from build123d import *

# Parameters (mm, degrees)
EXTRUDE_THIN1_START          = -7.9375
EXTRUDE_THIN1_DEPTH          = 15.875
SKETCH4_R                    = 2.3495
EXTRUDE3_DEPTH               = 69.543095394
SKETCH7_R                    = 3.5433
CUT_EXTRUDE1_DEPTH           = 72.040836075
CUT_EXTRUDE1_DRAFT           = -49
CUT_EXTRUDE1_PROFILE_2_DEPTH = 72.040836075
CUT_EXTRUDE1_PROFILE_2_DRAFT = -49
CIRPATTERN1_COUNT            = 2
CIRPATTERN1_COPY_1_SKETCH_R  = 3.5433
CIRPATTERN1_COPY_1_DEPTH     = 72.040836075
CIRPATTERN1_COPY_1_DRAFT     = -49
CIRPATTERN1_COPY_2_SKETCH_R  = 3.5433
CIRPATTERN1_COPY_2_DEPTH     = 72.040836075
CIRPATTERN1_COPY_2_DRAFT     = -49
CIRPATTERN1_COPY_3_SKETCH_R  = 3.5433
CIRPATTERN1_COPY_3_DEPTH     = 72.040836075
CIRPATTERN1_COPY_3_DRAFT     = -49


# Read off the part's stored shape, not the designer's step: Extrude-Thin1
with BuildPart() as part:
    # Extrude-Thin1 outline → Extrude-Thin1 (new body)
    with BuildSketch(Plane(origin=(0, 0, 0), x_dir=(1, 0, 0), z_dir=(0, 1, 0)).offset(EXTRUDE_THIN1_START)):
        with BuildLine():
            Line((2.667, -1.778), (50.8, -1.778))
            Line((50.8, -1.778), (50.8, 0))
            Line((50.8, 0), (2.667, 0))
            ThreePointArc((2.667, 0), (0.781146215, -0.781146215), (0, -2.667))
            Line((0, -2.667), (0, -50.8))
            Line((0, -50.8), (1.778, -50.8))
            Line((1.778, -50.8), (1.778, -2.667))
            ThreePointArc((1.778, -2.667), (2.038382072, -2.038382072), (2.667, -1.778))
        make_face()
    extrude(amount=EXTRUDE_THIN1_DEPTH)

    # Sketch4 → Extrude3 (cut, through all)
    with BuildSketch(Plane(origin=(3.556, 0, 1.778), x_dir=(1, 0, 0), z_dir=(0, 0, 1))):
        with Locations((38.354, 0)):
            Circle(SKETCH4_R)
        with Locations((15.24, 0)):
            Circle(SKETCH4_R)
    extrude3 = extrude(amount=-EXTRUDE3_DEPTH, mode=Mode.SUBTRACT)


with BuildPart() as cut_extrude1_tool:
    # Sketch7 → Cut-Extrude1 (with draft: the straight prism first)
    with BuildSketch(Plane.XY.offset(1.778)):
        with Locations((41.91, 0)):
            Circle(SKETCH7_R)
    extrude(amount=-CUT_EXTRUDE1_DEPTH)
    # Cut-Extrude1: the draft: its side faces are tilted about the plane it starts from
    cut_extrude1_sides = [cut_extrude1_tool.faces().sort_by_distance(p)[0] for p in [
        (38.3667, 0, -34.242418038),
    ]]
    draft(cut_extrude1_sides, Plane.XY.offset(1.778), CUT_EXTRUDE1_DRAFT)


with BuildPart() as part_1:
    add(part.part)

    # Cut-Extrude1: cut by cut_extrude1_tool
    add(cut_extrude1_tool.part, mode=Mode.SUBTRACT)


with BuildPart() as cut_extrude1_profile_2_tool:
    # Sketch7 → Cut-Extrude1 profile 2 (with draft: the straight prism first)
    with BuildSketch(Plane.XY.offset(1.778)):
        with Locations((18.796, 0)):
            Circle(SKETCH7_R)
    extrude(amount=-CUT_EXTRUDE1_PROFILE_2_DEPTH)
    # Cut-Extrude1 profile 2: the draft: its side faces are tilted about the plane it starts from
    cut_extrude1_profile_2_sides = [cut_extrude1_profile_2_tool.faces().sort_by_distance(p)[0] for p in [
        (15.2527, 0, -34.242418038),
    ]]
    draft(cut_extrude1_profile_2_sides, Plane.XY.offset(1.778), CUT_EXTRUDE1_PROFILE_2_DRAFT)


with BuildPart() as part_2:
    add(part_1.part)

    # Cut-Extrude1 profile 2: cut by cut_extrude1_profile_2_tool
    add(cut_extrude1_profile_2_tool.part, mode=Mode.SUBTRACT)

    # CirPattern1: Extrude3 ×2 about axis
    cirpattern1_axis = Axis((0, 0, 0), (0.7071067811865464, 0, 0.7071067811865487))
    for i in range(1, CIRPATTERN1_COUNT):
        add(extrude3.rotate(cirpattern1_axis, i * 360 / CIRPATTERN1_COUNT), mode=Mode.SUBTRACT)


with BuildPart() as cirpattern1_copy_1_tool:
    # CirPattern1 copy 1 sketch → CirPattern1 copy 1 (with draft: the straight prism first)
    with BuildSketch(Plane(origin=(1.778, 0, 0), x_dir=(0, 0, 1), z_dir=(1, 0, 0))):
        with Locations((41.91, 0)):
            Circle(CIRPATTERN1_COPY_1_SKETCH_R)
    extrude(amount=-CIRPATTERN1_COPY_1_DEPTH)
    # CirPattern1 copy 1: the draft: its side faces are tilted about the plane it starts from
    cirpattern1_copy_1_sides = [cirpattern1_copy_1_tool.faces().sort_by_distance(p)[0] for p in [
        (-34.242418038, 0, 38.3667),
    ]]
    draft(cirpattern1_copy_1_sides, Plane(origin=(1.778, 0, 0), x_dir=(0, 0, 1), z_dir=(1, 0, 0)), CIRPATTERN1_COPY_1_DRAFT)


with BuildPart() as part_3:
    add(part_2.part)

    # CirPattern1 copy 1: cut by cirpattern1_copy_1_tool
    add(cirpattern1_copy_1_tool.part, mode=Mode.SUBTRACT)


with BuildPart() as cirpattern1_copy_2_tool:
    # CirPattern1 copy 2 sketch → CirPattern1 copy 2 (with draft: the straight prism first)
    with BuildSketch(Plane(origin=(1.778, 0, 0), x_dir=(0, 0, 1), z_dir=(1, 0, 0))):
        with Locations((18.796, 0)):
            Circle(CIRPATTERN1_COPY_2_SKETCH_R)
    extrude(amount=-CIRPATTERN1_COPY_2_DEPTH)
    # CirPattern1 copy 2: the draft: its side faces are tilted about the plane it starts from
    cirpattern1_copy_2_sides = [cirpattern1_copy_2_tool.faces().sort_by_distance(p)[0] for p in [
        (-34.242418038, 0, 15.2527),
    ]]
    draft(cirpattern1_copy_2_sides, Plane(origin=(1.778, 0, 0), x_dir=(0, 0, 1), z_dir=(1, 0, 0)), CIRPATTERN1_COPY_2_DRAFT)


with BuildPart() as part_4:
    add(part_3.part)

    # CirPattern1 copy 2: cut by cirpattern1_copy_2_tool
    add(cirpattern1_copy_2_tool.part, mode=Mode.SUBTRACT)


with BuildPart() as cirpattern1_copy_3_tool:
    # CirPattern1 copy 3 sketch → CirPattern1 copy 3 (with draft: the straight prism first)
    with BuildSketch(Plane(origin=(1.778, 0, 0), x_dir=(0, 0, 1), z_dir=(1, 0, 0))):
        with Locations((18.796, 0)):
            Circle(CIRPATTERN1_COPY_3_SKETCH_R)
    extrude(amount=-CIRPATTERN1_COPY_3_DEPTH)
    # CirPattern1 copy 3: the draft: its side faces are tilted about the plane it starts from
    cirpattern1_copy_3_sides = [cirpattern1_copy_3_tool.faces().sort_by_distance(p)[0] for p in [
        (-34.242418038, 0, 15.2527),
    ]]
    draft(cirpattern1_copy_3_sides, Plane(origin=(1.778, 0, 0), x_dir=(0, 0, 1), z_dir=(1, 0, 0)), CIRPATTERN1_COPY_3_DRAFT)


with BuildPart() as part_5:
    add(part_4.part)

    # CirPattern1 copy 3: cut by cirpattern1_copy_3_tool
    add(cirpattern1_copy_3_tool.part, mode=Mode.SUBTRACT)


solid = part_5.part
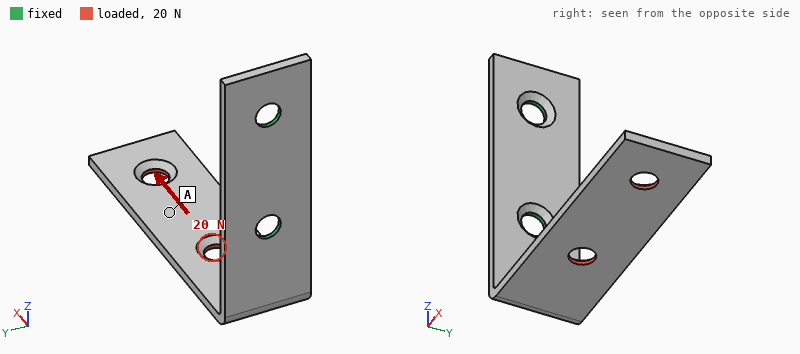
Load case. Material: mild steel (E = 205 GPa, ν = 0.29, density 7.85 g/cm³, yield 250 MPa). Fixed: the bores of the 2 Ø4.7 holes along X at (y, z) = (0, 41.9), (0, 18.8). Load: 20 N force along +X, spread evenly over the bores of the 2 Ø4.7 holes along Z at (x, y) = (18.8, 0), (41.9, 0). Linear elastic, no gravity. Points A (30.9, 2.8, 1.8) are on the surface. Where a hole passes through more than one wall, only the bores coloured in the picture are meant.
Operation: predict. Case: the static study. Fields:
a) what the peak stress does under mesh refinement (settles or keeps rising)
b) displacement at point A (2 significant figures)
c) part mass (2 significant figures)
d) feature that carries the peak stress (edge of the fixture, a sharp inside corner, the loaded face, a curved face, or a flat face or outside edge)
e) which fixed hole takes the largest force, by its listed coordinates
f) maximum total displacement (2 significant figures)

keeps rising
0.077 mm
21 g
edge of the fixture
(0, 18.8)
0.13 mm
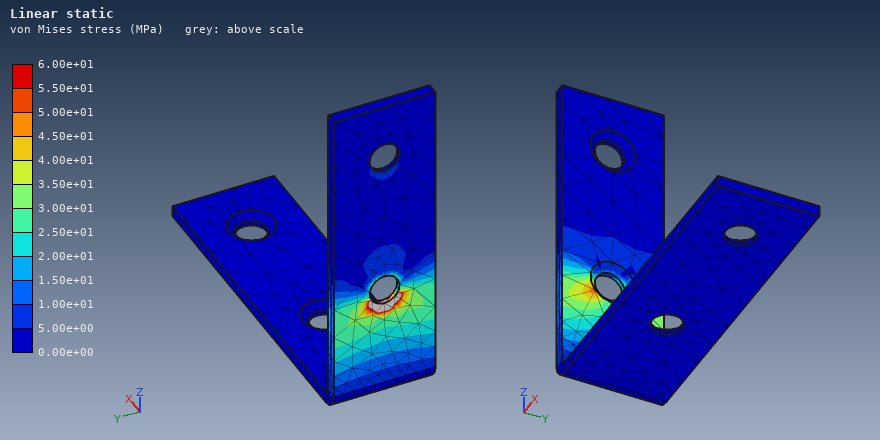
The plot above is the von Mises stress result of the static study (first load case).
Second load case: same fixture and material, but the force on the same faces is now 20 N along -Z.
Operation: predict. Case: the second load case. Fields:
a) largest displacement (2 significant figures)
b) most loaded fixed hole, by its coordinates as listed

0.60 mm
(0, 41.9)
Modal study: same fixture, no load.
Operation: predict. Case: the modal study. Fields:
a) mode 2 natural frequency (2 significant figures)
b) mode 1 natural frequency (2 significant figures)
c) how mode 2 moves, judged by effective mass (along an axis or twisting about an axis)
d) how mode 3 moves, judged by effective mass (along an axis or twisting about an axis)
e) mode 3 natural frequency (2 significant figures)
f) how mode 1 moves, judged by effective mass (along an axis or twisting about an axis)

620 Hz
380 Hz
along Y
along X
1700 Hz
along Z
